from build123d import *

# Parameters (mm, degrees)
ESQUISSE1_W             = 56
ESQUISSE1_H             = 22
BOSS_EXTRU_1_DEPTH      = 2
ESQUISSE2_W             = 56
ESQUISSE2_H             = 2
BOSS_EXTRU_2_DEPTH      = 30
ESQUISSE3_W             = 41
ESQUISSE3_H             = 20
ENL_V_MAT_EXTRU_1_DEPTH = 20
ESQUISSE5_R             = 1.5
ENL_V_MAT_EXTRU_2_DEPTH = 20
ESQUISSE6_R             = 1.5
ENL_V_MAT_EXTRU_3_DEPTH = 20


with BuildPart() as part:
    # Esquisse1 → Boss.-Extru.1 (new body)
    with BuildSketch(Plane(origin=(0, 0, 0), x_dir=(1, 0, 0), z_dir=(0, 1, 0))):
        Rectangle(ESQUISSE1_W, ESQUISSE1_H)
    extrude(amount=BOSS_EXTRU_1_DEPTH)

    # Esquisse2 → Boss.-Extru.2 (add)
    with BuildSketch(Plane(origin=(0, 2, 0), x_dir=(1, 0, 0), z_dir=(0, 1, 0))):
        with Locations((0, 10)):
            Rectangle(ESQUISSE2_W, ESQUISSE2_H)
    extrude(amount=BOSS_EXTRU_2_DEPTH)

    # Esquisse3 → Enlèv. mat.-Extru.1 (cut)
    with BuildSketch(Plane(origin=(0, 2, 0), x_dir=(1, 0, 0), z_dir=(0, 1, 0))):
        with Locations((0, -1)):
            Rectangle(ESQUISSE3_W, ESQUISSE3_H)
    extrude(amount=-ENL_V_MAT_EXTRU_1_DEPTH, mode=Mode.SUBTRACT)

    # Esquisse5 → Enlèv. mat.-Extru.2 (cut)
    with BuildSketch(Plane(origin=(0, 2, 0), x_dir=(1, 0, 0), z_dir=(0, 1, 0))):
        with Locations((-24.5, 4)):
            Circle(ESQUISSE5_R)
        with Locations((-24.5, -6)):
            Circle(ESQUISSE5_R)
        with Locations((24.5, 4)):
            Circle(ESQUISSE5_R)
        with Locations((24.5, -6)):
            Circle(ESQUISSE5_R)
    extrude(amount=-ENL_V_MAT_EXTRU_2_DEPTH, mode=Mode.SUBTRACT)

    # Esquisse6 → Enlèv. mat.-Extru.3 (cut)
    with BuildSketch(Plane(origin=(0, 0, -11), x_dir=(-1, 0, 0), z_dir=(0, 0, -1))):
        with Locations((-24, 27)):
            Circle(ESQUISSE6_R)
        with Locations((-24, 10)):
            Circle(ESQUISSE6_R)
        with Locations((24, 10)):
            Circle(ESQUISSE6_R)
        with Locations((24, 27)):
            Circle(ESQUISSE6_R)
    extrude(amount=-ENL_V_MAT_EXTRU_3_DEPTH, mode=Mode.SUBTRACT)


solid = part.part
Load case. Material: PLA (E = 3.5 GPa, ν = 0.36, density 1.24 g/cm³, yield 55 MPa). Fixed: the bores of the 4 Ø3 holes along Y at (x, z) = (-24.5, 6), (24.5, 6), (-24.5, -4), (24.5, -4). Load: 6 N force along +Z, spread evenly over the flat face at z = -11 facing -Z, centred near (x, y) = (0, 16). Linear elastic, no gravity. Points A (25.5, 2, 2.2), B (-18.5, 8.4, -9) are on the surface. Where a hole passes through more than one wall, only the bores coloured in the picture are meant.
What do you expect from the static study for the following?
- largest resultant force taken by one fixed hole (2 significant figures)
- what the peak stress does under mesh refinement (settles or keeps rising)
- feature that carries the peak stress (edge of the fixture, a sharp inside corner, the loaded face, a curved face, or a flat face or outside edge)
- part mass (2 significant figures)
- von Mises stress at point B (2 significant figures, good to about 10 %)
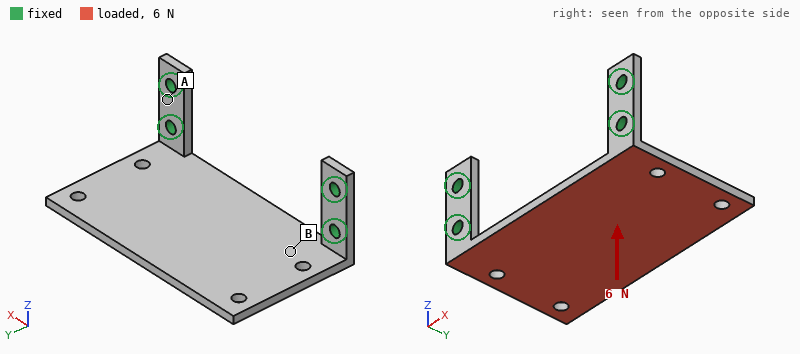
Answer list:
2.9 N
keeps rising
edge of the fixture
5.0 g
2.1 MPa
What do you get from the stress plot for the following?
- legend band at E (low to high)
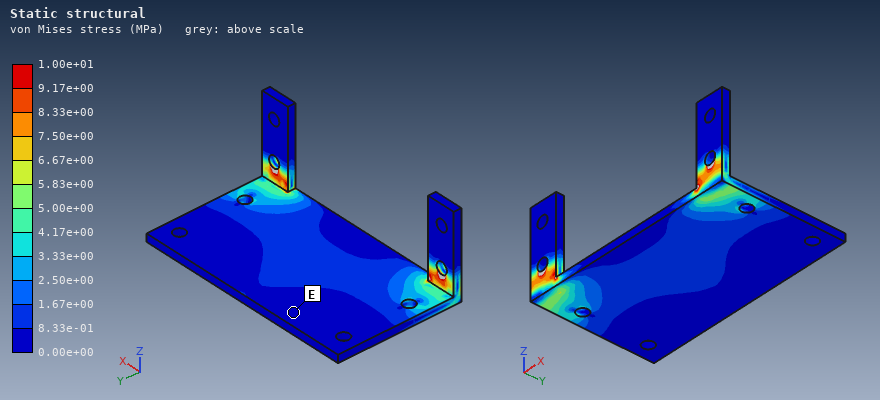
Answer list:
0.00e+00 to 8.33e-01 MPa
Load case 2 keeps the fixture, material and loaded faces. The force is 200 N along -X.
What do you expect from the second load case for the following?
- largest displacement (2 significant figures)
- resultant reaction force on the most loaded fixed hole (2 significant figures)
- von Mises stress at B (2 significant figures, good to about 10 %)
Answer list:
0.30 mm
130 N
7.5 MPa
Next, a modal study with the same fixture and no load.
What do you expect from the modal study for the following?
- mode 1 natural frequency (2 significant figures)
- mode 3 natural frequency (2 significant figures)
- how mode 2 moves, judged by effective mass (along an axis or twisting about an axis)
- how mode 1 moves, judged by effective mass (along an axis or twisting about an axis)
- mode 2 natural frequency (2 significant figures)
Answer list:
270 Hz
1400 Hz
twisting about Y
along Z
760 Hz
